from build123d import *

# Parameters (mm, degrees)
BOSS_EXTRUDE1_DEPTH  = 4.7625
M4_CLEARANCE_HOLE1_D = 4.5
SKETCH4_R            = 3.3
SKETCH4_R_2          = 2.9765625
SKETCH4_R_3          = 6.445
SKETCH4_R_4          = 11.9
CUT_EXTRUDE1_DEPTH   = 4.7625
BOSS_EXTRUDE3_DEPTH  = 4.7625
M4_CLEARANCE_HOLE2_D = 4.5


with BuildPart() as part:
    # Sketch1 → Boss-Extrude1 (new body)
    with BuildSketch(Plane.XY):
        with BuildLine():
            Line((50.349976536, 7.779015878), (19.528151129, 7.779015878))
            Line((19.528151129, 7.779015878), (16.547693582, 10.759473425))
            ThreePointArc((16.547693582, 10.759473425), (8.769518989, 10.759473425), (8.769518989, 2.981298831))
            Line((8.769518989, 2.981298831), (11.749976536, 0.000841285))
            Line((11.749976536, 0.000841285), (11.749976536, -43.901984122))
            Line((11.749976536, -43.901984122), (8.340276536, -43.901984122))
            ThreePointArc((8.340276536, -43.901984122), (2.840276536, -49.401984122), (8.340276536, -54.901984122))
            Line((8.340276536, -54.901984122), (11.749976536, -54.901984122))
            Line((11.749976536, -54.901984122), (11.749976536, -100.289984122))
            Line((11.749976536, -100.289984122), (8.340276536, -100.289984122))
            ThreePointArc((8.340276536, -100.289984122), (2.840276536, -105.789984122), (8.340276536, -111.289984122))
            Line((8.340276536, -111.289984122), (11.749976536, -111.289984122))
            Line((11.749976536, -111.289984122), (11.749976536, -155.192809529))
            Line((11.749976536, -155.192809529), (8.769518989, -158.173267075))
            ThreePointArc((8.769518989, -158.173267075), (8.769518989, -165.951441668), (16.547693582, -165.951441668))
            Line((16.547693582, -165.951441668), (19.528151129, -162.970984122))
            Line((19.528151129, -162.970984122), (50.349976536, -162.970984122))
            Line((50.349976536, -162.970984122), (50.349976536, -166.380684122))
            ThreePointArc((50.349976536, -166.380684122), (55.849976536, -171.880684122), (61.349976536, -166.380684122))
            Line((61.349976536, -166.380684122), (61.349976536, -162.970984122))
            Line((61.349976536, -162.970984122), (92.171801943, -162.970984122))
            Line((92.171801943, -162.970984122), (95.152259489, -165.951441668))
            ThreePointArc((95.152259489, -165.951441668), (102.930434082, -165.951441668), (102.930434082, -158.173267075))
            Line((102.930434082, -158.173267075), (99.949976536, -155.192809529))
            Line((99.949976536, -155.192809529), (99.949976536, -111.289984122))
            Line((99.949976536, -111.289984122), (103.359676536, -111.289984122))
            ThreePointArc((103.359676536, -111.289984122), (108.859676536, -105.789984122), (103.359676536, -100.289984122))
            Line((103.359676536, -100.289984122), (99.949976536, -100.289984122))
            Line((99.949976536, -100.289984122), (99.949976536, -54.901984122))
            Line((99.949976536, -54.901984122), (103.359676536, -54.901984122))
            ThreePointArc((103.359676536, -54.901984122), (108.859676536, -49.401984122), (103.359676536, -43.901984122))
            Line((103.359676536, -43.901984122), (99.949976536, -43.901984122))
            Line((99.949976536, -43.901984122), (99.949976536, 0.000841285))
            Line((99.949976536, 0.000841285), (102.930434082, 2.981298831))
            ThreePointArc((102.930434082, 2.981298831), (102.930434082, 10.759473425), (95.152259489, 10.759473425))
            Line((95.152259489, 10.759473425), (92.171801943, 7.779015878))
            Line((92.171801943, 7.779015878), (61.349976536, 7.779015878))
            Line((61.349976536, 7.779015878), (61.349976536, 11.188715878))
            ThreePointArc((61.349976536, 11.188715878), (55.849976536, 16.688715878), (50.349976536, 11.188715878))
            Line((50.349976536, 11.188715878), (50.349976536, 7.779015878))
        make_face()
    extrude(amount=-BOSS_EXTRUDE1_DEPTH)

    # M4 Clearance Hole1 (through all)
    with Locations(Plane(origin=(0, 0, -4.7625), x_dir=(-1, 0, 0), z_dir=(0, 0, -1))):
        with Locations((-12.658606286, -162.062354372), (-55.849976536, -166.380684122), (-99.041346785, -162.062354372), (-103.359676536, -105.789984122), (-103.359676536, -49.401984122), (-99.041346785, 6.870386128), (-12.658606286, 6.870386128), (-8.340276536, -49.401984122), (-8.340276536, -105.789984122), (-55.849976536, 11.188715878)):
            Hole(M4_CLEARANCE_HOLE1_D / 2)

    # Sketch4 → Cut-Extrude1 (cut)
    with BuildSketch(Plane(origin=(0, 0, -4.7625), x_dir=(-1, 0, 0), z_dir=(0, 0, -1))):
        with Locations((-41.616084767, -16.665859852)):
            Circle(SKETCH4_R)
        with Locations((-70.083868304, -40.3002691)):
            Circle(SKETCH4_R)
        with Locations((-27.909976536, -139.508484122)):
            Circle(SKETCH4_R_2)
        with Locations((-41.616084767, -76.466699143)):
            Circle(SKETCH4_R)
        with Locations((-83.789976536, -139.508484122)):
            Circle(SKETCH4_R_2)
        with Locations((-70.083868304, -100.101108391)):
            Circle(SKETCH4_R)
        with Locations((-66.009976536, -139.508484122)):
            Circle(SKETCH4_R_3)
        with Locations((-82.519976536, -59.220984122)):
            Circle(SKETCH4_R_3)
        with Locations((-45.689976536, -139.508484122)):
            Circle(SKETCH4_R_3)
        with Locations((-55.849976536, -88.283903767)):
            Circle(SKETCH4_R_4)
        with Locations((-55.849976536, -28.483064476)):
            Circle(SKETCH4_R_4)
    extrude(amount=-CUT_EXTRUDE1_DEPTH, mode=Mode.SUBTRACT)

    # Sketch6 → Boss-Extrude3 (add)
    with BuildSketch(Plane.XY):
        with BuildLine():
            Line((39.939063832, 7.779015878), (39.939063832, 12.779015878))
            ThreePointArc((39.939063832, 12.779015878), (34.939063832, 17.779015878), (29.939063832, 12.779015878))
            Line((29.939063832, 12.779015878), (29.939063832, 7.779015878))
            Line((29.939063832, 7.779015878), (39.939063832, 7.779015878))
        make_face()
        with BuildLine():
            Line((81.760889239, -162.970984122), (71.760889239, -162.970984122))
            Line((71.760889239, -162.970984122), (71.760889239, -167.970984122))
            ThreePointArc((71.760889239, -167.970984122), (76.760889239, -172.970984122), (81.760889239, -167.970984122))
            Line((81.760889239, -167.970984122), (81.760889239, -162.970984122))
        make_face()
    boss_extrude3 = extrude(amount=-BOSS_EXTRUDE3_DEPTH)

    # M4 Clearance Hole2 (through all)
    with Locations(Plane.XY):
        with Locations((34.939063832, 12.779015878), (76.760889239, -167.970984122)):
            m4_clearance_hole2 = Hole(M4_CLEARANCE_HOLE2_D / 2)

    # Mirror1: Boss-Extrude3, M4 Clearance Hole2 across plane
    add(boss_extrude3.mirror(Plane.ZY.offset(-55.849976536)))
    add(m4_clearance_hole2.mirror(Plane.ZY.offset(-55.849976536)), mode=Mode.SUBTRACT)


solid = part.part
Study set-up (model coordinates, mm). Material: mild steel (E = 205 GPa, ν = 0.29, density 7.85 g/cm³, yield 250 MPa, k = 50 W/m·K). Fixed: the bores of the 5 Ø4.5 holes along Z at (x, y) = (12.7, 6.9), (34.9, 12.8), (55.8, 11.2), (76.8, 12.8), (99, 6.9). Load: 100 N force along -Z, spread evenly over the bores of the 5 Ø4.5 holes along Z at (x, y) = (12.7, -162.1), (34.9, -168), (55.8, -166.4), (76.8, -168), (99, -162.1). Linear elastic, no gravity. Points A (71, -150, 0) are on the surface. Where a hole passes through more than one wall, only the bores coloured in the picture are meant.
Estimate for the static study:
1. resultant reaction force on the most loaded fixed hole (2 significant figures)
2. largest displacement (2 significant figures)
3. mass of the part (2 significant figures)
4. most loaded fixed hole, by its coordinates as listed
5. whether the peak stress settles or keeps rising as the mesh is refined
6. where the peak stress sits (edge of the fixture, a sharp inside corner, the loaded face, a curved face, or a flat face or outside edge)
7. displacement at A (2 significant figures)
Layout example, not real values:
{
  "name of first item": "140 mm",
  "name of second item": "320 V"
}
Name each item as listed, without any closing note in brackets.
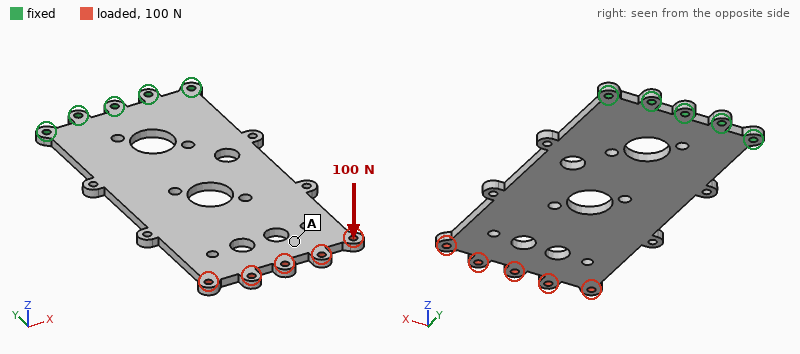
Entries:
{
  "resultant reaction force on the most loaded fixed hole": "130 N",
  "largest displacement": "1.4 mm",
  "mass of the part": "540 g",
  "most loaded fixed hole, by its coordinates as listed": "(55.8, 11.2)",
  "whether the peak stress settles or keeps rising as the mesh is refined": "keeps rising",
  "where the peak stress sits": "edge of the fixture",
  "displacement at A": "1.2 mm"
}
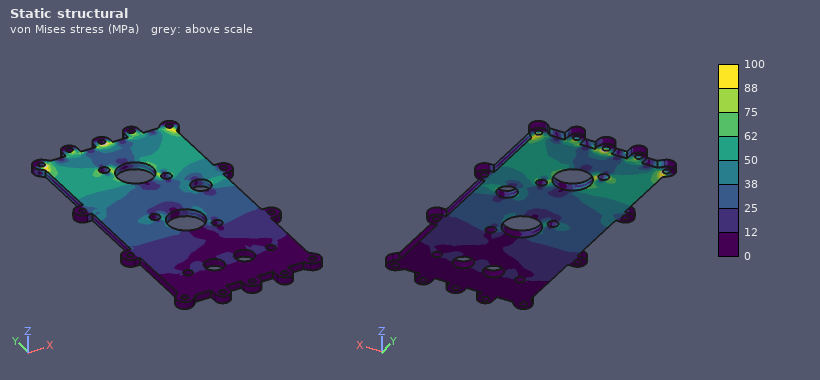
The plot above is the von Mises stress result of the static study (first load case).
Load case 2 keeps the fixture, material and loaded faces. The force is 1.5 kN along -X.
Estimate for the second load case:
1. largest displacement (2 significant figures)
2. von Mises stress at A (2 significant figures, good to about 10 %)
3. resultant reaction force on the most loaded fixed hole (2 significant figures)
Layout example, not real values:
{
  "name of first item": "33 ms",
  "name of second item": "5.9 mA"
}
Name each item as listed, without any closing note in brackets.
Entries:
{
  "largest displacement": "72 µm",
  "von Mises stress at A": "11 MPa",
  "resultant reaction force on the most loaded fixed hole": "2.6 kN"
}
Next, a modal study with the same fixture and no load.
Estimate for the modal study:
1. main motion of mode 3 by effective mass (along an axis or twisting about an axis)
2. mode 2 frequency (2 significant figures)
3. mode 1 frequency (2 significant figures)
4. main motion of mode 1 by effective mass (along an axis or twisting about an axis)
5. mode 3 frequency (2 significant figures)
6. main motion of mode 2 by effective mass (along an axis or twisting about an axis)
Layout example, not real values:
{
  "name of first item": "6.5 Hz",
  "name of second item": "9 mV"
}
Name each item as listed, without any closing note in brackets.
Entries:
{
  "main motion of mode 3 by effective mass": "along Z",
  "mode 2 frequency": "500 Hz",
  "mode 1 frequency": "120 Hz",
  "main motion of mode 1 by effective mass": "along Z",
  "mode 3 frequency": "740 Hz",
  "main motion of mode 2 by effective mass": "twisting about Y"
}
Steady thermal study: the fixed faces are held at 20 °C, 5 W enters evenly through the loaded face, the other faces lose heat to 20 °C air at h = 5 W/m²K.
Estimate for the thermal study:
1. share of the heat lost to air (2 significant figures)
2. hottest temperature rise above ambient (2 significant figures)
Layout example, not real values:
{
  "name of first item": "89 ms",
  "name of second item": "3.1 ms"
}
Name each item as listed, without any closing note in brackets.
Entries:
{
  "share of the heat lost to air": "51 %",
  "hottest temperature rise above ambient": "35 K"
}
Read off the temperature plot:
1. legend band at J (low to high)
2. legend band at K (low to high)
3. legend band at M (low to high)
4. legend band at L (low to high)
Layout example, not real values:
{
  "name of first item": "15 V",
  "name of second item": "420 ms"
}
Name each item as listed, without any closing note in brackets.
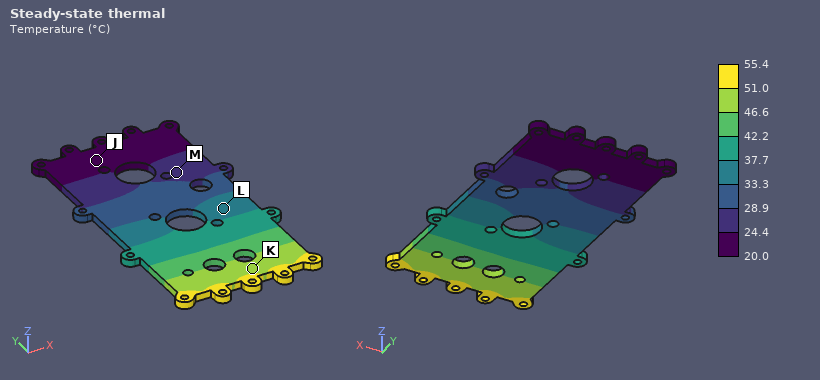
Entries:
{
  "legend band at J": "20.0 to 24.4 °C",
  "legend band at K": "46.6 to 51.0 °C",
  "legend band at M": "24.4 to 28.9 °C",
  "legend band at L": "33.3 to 37.7 °C"
}
